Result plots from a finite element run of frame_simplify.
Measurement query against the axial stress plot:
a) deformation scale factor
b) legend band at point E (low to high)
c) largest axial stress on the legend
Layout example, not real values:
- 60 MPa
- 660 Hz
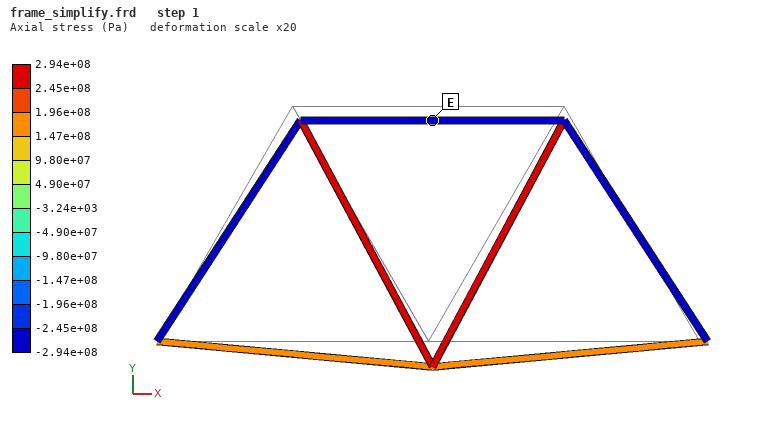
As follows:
- 20
- -2.94e+08 to -2.45e+08 Pa
- 2.94e+08 Pa
